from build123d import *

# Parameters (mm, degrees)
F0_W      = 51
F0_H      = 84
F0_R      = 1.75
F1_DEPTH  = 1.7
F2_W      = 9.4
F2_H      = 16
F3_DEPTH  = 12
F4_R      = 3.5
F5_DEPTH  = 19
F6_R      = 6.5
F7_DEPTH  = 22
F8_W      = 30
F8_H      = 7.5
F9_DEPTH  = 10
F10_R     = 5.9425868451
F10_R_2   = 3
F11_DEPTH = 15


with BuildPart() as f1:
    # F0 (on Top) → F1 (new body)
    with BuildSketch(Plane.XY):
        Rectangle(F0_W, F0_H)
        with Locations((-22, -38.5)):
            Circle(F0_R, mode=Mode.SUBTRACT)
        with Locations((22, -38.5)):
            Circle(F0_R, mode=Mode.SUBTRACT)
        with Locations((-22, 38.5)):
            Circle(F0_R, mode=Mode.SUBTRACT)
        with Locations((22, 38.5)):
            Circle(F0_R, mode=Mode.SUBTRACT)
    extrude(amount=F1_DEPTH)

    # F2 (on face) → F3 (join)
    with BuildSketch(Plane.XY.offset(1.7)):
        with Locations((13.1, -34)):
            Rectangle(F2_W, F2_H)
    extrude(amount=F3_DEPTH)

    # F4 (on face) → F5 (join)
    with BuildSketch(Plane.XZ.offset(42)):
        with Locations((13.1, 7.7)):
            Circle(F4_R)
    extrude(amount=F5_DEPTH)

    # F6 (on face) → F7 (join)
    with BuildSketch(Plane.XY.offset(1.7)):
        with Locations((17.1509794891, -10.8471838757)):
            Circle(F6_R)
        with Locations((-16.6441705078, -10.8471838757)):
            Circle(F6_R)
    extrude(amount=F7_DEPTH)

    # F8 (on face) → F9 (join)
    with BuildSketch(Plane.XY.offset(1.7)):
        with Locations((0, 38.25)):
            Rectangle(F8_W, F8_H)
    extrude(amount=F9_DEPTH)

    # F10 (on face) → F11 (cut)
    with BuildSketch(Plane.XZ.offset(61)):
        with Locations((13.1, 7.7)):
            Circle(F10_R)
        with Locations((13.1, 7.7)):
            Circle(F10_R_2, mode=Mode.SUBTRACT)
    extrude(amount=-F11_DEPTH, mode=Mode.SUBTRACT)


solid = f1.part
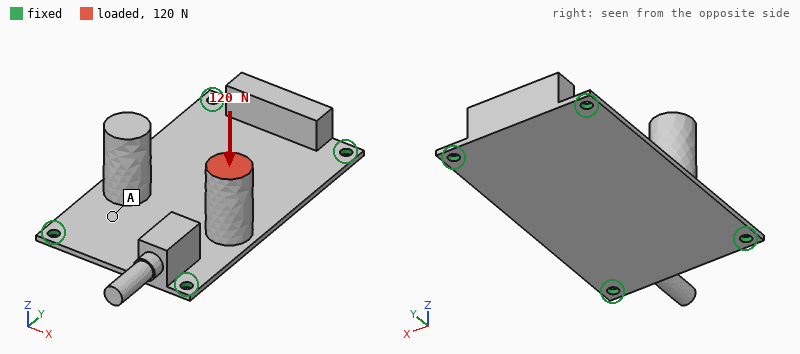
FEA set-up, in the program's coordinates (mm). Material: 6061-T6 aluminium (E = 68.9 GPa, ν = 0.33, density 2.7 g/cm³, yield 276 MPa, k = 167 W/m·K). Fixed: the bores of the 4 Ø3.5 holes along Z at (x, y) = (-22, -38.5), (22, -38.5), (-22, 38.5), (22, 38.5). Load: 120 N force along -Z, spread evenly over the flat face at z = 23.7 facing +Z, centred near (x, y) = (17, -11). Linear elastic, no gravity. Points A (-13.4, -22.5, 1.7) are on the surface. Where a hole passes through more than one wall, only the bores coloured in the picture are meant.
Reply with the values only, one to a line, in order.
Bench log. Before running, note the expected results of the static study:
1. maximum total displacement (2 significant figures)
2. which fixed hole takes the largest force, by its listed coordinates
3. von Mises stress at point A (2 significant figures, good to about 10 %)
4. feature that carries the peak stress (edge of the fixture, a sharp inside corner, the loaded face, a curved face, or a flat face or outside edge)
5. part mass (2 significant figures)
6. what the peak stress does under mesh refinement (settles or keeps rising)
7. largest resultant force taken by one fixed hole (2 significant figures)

0.23 mm
(22, -38.5)
7.8 MPa
edge of the fixture
48 g
keeps rising
80 N
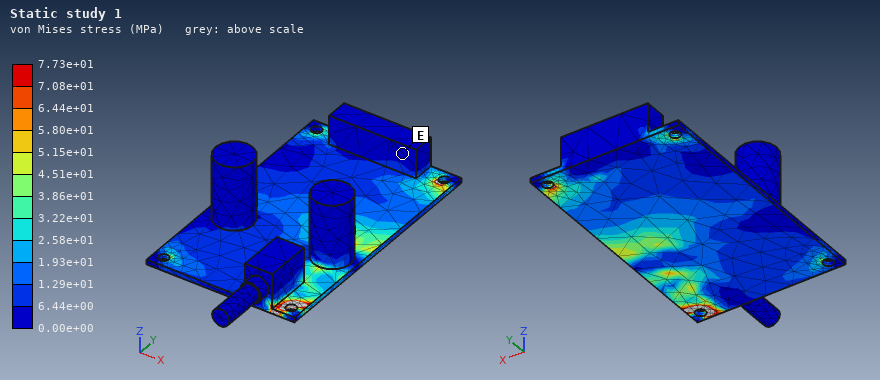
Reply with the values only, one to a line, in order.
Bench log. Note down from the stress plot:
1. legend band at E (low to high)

0.00e+00 to 6.44e+00 MPa
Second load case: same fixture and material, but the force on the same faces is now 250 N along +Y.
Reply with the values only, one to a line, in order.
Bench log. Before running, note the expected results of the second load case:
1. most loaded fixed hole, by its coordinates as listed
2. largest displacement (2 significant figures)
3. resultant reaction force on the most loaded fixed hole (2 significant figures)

(22, -38.5)
0.65 mm
140 N
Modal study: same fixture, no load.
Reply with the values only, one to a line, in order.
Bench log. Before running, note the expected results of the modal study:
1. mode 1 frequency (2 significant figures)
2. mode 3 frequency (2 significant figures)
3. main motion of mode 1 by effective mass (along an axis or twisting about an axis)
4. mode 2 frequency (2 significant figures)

920 Hz
1500 Hz
along Z
1200 Hz
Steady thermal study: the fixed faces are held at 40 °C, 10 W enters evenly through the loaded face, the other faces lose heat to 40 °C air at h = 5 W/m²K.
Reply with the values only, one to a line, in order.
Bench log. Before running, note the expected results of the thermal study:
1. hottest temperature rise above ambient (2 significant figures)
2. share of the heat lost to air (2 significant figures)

29 K
5.0 %
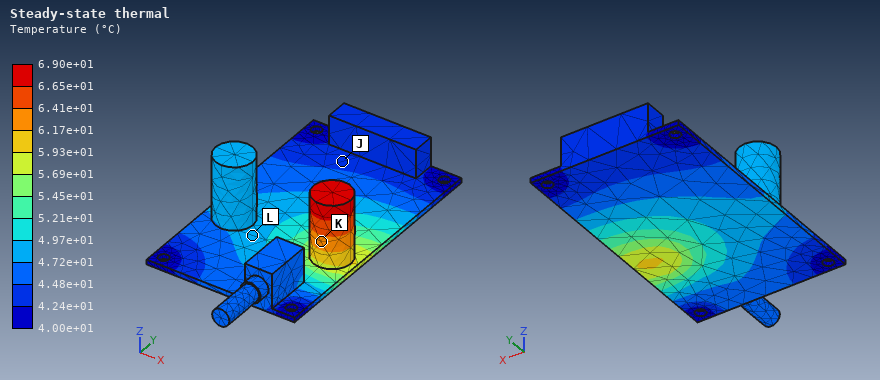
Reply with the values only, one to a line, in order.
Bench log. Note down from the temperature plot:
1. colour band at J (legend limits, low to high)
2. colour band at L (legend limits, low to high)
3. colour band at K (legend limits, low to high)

4.24e+01 to 4.48e+01 °C
4.72e+01 to 4.97e+01 °C
6.17e+01 to 6.41e+01 °C
